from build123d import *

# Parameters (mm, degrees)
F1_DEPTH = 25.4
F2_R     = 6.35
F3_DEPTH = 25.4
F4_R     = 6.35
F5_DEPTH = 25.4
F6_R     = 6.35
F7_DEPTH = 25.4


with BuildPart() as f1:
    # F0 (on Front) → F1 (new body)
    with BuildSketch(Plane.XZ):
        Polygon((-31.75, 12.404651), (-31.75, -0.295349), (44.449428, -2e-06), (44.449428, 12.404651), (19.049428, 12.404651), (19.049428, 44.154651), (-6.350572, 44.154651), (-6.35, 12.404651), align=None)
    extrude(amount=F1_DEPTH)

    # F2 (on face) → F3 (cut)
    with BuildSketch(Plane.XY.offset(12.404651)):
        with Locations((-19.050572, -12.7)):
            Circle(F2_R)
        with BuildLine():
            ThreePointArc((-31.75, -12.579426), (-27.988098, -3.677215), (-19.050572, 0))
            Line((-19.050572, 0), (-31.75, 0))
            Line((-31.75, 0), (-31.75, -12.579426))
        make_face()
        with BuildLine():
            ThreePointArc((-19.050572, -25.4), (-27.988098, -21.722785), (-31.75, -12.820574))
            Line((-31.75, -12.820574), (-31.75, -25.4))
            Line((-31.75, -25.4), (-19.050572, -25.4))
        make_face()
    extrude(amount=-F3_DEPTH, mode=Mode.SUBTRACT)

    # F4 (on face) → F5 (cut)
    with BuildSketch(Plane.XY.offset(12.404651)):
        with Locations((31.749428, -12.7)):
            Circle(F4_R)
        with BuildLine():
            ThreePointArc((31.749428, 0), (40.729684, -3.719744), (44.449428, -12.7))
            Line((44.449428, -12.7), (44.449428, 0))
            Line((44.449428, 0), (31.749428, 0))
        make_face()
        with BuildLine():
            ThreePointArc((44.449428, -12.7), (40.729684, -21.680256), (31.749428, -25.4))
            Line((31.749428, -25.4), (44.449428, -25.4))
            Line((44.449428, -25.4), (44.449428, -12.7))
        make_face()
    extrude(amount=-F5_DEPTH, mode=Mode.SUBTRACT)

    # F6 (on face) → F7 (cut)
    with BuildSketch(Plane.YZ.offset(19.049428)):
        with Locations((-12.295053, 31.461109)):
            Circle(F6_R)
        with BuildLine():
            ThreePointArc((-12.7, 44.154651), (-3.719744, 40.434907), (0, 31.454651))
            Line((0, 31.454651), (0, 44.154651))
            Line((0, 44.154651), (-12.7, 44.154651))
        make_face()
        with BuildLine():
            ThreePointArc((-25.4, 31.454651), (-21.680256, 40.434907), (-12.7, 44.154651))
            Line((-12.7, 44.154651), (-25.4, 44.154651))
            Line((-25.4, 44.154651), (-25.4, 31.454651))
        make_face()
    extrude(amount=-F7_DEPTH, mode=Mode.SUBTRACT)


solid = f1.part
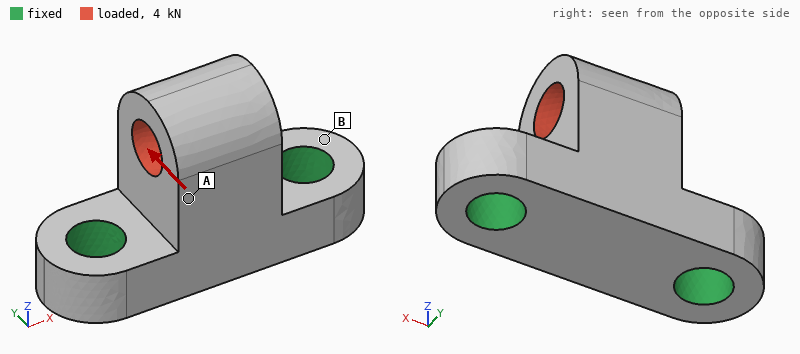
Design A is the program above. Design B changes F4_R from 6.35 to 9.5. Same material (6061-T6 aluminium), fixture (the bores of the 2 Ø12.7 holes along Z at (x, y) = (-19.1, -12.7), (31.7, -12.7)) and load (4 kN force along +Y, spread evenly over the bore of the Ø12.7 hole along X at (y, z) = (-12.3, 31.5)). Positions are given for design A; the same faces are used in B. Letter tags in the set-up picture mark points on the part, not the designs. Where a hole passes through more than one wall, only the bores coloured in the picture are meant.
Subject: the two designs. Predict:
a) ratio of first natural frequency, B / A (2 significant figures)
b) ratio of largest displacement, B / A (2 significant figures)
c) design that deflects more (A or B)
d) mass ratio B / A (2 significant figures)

1.1
0.85
A
0.94
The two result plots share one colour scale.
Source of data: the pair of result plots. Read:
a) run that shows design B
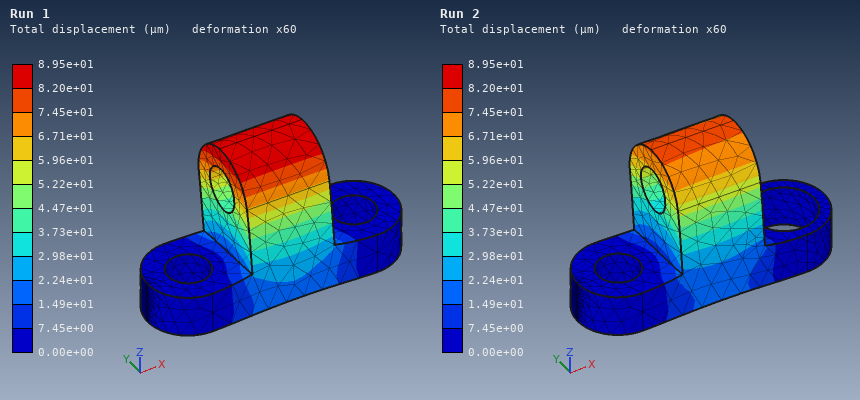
Run 2
